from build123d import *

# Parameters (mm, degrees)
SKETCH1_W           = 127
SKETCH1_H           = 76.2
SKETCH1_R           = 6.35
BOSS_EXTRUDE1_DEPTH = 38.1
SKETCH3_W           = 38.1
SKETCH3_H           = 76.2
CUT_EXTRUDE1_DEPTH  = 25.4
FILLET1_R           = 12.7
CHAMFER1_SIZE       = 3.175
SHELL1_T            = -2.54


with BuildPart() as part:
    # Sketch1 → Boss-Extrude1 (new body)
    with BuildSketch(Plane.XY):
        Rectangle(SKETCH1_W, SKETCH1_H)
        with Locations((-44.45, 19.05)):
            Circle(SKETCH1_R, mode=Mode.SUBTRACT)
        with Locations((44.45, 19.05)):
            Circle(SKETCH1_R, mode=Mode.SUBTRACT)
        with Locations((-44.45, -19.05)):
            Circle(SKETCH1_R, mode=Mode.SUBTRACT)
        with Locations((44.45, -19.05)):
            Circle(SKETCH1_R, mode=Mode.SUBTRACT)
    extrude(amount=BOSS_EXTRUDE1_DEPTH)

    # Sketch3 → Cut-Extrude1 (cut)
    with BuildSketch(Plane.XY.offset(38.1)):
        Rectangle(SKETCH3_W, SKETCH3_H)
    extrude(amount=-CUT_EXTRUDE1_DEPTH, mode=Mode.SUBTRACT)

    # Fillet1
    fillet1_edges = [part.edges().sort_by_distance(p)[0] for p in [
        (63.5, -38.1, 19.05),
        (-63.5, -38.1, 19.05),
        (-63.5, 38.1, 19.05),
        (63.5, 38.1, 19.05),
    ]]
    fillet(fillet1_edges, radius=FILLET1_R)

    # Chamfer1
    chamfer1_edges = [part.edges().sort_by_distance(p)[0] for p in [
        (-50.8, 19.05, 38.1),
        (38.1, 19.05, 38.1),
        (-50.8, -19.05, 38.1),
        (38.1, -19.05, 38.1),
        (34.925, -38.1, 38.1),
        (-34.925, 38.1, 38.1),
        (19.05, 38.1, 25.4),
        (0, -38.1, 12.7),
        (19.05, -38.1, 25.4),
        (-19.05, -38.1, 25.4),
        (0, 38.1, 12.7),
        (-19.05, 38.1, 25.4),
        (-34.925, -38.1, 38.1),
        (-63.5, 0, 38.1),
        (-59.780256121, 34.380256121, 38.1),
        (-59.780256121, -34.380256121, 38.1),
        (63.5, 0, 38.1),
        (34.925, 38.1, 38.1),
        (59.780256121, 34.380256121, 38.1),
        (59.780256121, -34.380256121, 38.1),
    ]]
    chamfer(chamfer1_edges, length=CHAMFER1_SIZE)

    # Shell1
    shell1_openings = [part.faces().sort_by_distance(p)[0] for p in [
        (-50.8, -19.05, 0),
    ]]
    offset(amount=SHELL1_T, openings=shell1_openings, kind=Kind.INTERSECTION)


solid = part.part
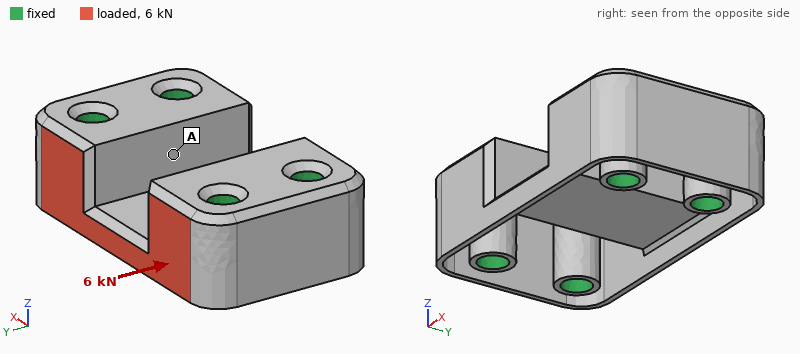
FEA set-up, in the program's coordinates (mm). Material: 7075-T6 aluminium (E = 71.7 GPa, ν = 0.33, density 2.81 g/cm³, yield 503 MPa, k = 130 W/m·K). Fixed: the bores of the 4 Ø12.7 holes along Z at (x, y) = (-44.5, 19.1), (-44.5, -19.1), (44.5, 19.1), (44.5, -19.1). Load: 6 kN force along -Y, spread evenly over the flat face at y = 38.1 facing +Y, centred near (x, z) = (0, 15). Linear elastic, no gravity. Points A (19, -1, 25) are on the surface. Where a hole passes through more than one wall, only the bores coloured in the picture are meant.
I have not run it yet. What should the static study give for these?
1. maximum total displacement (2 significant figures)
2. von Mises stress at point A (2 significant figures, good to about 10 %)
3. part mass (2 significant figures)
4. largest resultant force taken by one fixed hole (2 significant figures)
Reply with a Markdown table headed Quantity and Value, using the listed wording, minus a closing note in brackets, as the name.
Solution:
| Quantity | Value |
|---|---|
| maximum total displacement | 0.44 mm |
| von Mises stress at point A | 21 MPa |
| part mass | 210 g |
| largest resultant force taken by one fixed hole | 2.2 kN |
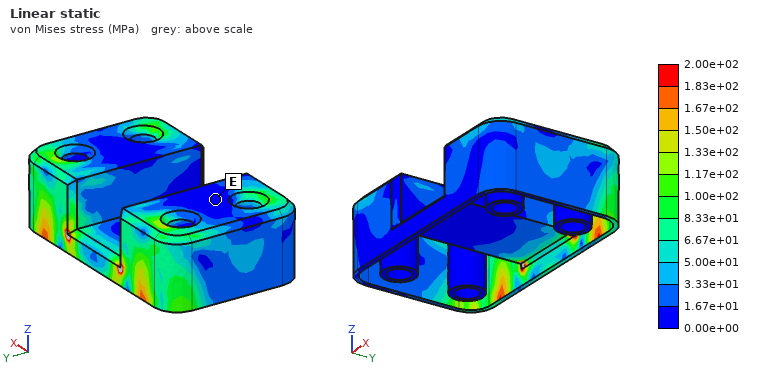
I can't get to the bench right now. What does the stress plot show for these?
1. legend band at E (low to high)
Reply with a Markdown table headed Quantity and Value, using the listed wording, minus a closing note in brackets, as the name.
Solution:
| Quantity | Value |
|---|---|
| legend band at E | 0.00e+00 to 1.67e+01 MPa |
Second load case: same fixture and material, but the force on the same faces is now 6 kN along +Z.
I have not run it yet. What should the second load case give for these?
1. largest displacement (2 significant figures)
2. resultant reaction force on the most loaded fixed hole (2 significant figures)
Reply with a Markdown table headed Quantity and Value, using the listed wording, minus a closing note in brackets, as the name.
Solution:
| Quantity | Value |
|---|---|
| largest displacement | 0.31 mm |
| resultant reaction force on the most loaded fixed hole | 3.9 kN |
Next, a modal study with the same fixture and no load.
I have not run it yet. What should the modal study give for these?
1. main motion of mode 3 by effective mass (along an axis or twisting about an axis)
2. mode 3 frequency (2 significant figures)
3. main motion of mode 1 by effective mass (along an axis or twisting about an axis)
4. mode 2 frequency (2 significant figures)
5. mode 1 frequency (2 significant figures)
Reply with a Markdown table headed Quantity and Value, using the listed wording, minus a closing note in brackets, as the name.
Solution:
| Quantity | Value |
|---|---|
| main motion of mode 3 by effective mass | along Y |
| mode 3 frequency | 3100 Hz |
| main motion of mode 1 by effective mass | along X |
| mode 2 frequency | 2800 Hz |
| mode 1 frequency | 2700 Hz |
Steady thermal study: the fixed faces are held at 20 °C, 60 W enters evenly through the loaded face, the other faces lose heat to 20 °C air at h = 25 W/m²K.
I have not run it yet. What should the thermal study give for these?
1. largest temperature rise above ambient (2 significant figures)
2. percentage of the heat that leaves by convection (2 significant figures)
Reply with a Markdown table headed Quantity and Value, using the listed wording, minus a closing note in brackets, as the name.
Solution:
| Quantity | Value |
|---|---|
| largest temperature rise above ambient | 39 K |
| percentage of the heat that leaves by convection | 20 % |
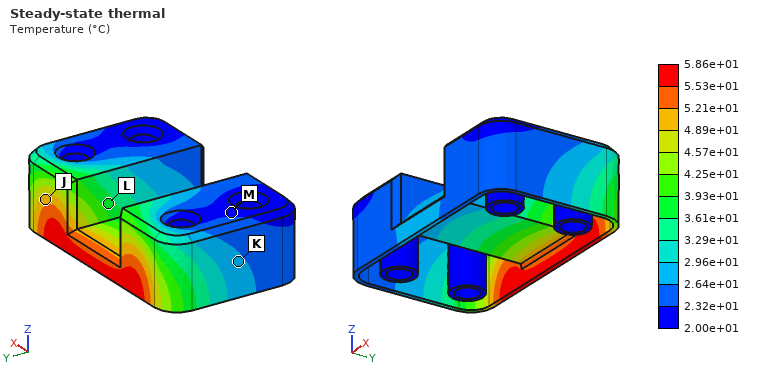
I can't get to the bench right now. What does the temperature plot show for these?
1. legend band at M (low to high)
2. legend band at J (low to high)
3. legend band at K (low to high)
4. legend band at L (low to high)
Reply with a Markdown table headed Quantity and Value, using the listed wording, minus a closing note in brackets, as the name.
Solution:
| Quantity | Value |
|---|---|
| legend band at M | 2.00e+01 to 2.32e+01 °C |
| legend band at J | 4.89e+01 to 5.21e+01 °C |
| legend band at K | 2.64e+01 to 2.96e+01 °C |
| legend band at L | 3.61e+01 to 3.93e+01 °C |
